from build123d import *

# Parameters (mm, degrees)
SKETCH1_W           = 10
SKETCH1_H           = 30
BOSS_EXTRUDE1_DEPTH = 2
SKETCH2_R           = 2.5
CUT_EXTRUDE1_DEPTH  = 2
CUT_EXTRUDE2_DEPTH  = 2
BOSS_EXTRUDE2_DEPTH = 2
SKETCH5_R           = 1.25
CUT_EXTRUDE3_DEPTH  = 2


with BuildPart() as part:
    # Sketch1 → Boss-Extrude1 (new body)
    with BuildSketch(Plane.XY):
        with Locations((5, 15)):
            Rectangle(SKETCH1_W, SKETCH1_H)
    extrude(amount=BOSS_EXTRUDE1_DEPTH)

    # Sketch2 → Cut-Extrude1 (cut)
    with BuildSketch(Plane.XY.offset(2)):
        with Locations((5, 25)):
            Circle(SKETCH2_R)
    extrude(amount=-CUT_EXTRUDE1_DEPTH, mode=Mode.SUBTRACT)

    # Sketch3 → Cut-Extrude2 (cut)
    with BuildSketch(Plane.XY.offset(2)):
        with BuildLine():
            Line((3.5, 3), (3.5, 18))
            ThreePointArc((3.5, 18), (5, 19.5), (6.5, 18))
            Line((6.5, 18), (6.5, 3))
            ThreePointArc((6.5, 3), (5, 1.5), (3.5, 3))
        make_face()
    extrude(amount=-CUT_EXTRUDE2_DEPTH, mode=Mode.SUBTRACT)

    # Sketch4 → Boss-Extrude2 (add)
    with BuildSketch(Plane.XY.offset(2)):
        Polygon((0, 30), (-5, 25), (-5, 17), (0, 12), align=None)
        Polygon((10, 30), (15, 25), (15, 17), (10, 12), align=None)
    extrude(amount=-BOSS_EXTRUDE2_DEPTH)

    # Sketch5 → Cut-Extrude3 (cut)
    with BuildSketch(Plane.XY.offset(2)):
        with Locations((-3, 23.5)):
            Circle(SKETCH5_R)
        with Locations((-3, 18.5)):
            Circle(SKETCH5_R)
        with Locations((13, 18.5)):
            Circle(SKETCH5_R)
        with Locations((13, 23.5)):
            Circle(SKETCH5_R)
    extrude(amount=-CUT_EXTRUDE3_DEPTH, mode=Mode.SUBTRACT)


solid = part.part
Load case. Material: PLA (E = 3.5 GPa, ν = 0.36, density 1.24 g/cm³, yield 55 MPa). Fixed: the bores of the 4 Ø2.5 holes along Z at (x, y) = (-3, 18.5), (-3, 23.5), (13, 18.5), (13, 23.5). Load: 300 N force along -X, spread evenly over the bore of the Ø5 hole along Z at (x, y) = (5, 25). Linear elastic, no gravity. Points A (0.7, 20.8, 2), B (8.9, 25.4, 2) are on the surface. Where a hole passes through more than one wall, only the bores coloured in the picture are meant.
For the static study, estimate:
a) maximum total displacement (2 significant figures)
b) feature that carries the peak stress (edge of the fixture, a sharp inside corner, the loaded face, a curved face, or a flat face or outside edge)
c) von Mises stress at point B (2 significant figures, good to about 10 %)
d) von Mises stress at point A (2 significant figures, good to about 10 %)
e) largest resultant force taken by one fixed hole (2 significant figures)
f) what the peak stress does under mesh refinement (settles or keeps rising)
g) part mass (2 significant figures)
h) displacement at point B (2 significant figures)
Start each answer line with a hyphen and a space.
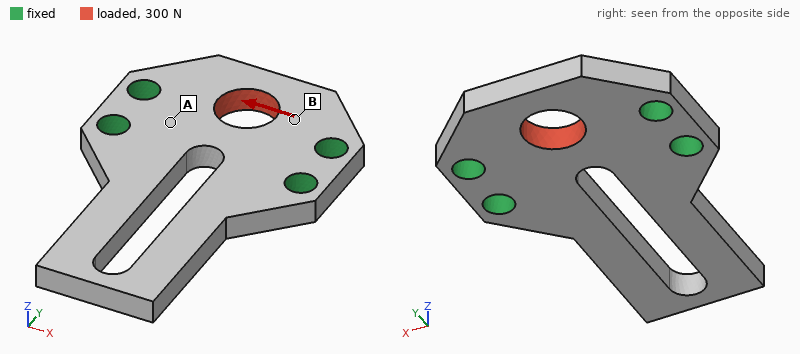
- 38 µm
- edge of the fixture
- 15 MPa
- 4.7 MPa
- 130 N
- keeps rising
- 0.84 g
- 19 µm
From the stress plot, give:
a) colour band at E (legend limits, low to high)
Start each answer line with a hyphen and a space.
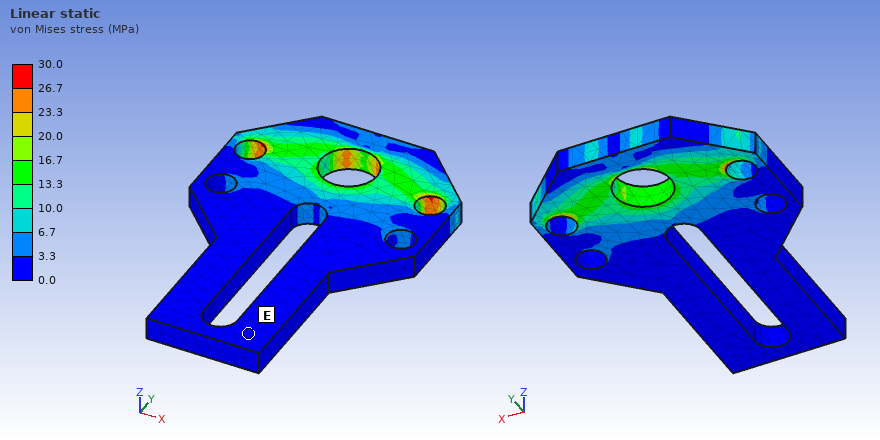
- 0.0 to 3.3 MPa
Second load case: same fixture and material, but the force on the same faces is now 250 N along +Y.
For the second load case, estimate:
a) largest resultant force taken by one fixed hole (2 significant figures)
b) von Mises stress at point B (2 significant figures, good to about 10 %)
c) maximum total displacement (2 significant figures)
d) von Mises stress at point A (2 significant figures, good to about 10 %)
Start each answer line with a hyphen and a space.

- 76 N
- 12 MPa
- 44 µm
- 9.6 MPa
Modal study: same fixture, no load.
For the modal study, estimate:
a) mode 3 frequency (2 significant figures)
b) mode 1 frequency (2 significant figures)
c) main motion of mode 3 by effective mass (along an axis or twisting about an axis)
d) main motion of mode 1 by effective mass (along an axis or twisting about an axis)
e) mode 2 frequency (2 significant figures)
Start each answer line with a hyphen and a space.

- 5900 Hz
- 1700 Hz
- along X
- along Z
- 5200 Hz
